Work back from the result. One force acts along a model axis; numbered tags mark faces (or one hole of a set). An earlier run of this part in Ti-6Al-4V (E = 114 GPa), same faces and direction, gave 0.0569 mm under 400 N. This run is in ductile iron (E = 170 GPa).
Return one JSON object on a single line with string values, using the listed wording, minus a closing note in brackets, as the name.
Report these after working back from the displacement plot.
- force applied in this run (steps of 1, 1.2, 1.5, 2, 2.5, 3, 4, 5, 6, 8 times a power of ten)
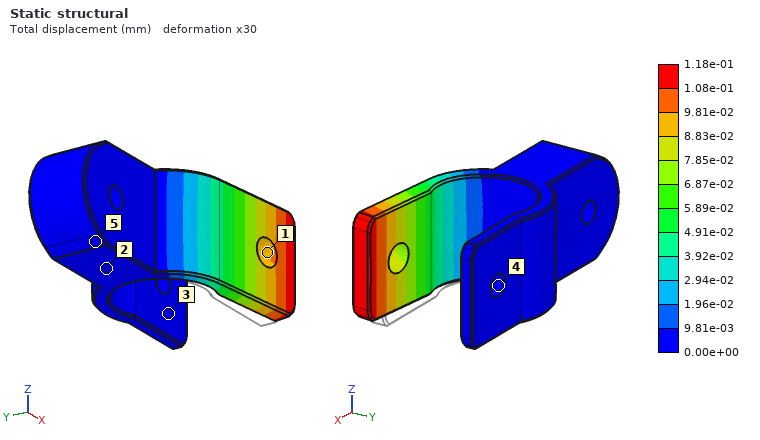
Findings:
{"force applied in this run": "1.2 kN"}
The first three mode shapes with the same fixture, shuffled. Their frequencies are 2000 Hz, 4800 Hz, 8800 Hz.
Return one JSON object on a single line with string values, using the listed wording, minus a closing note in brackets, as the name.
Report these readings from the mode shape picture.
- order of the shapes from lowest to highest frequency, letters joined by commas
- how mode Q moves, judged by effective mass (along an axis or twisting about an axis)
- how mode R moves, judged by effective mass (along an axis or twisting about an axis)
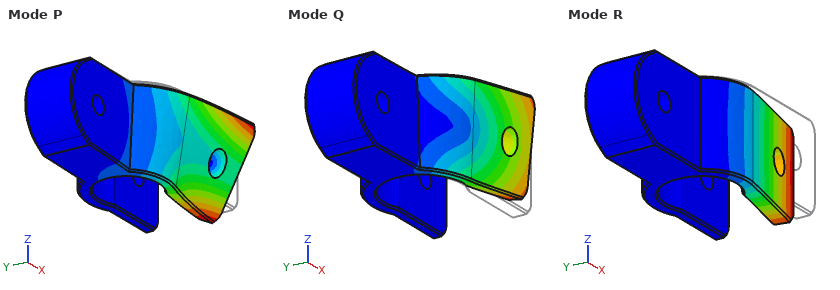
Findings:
{"order of the shapes from lowest to highest frequency, letters joined by commas": "R, Q, P", "how mode Q moves, judged by effective mass": "along Z", "how mode R moves, judged by effective mass": "along Y"}
